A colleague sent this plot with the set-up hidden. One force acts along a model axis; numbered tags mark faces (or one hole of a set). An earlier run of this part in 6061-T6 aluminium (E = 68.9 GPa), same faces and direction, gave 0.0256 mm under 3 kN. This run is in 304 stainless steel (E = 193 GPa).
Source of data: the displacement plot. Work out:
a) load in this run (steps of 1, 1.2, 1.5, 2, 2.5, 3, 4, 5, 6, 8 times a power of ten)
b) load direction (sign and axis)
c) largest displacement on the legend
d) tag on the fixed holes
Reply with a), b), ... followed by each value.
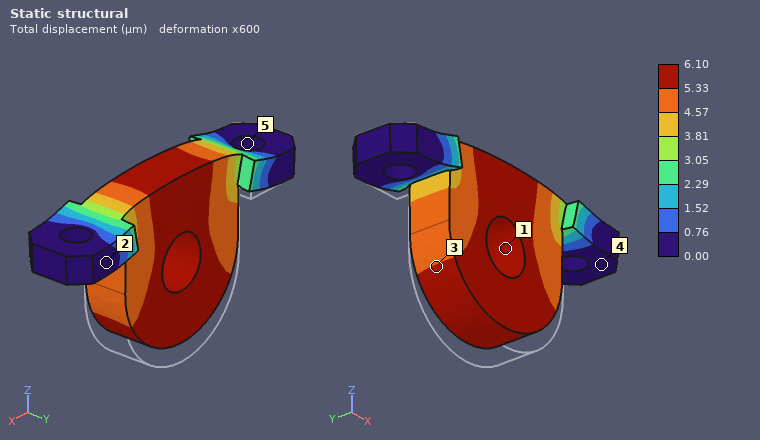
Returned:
a) 2 kN
b) +Z
c) 6.10 µm
d) 5
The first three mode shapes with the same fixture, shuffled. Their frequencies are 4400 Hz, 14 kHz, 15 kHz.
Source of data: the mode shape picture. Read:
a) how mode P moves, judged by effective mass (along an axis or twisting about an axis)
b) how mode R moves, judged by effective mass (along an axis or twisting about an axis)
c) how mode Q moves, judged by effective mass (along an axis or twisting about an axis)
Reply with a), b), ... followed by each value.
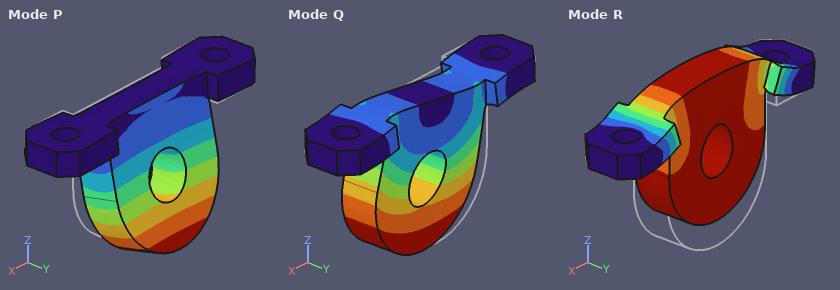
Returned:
a) along Y
b) along Z
c) along X
